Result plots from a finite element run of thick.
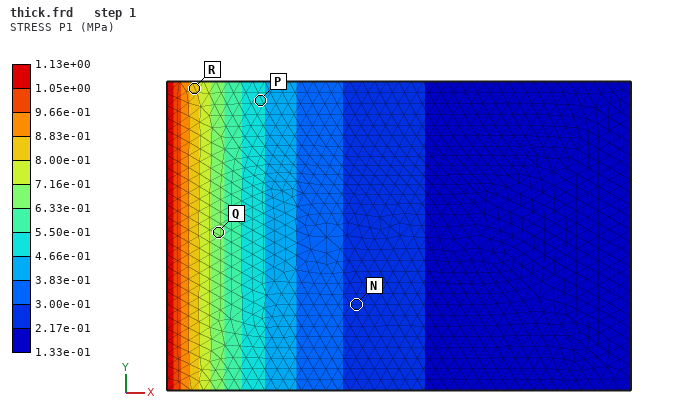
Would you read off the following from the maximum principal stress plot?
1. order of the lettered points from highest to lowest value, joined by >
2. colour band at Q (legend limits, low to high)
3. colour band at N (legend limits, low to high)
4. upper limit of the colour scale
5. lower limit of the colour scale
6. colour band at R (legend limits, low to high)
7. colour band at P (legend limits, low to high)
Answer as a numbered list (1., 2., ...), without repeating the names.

1. R > Q > P > N
2. 6.33e-01 to 7.16e-01 MPa
3. 2.17e-01 to 3.00e-01 MPa
4. 1.13e+00 MPa
5. 1.33e-01 MPa
6. 8.00e-01 to 8.83e-01 MPa
7. 4.66e-01 to 5.50e-01 MPa
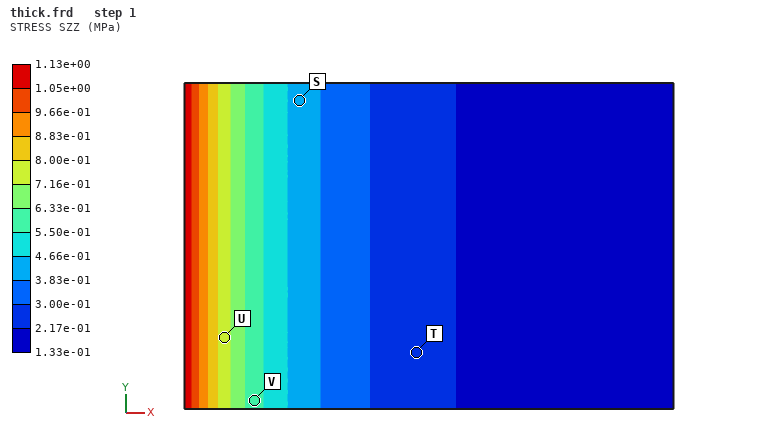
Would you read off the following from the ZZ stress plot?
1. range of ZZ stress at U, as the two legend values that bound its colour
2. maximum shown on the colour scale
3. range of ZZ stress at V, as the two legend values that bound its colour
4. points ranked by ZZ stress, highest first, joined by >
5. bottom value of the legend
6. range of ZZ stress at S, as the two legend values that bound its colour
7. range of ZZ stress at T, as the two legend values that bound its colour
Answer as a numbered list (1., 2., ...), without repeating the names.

1. 7.16e-01 to 8.00e-01 MPa
2. 1.13e+00 MPa
3. 5.50e-01 to 6.33e-01 MPa
4. U > V > S > T
5. 1.33e-01 MPa
6. 3.83e-01 to 4.66e-01 MPa
7. 2.17e-01 to 3.00e-01 MPa
